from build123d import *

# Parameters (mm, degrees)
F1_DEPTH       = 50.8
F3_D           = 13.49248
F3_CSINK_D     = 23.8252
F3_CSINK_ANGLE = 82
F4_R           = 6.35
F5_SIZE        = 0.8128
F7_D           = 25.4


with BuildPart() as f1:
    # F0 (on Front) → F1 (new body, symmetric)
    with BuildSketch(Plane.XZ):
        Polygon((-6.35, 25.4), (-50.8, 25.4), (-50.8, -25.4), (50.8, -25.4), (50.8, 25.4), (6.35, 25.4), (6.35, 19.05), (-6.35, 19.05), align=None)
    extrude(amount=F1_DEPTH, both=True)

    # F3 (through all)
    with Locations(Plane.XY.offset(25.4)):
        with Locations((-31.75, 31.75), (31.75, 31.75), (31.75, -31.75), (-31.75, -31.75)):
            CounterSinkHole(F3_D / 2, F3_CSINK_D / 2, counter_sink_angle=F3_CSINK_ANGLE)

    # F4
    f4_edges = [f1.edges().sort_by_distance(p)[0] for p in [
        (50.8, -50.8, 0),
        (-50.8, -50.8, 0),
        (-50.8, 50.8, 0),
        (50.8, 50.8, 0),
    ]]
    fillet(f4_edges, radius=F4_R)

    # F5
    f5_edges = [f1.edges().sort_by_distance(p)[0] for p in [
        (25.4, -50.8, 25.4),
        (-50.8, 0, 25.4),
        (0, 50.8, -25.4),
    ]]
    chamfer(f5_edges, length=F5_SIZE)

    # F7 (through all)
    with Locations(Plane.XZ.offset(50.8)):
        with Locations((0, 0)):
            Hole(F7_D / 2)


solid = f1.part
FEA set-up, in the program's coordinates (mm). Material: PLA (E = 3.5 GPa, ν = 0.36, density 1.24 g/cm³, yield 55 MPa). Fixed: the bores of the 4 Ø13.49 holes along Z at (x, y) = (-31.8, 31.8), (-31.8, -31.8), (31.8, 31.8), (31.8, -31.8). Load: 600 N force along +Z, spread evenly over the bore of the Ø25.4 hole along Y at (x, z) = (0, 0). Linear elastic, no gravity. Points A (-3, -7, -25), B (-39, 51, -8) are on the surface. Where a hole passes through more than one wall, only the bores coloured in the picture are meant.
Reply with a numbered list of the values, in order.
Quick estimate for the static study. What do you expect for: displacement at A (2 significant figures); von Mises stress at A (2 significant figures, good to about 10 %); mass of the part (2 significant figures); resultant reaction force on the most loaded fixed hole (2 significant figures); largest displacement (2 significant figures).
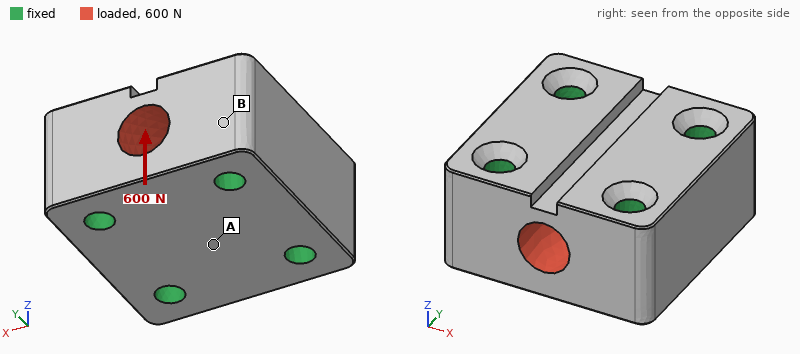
1. 1.9 µm
2. 0.16 MPa
3. 530 g
4. 150 N
5. 2.8 µm
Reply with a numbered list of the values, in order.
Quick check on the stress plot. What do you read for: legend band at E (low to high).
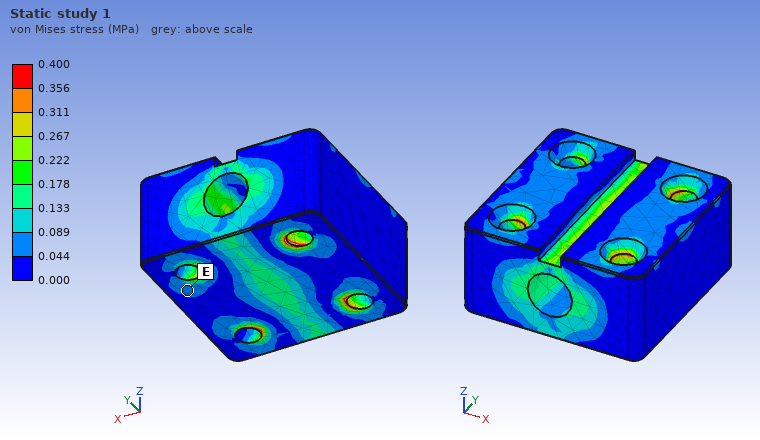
1. 0.044 to 0.089 MPa
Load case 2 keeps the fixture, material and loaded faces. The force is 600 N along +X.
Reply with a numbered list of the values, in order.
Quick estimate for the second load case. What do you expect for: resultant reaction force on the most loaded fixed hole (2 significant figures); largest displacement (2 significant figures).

1. 150 N
2. 0.97 µm
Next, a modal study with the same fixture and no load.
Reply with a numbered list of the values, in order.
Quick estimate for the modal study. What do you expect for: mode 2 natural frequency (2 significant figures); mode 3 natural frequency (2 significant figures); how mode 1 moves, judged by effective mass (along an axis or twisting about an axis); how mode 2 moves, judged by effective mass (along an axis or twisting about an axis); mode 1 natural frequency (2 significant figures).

1. 7200 Hz
2. 7600 Hz
3. along Z
4. along X
5. 6600 Hz
